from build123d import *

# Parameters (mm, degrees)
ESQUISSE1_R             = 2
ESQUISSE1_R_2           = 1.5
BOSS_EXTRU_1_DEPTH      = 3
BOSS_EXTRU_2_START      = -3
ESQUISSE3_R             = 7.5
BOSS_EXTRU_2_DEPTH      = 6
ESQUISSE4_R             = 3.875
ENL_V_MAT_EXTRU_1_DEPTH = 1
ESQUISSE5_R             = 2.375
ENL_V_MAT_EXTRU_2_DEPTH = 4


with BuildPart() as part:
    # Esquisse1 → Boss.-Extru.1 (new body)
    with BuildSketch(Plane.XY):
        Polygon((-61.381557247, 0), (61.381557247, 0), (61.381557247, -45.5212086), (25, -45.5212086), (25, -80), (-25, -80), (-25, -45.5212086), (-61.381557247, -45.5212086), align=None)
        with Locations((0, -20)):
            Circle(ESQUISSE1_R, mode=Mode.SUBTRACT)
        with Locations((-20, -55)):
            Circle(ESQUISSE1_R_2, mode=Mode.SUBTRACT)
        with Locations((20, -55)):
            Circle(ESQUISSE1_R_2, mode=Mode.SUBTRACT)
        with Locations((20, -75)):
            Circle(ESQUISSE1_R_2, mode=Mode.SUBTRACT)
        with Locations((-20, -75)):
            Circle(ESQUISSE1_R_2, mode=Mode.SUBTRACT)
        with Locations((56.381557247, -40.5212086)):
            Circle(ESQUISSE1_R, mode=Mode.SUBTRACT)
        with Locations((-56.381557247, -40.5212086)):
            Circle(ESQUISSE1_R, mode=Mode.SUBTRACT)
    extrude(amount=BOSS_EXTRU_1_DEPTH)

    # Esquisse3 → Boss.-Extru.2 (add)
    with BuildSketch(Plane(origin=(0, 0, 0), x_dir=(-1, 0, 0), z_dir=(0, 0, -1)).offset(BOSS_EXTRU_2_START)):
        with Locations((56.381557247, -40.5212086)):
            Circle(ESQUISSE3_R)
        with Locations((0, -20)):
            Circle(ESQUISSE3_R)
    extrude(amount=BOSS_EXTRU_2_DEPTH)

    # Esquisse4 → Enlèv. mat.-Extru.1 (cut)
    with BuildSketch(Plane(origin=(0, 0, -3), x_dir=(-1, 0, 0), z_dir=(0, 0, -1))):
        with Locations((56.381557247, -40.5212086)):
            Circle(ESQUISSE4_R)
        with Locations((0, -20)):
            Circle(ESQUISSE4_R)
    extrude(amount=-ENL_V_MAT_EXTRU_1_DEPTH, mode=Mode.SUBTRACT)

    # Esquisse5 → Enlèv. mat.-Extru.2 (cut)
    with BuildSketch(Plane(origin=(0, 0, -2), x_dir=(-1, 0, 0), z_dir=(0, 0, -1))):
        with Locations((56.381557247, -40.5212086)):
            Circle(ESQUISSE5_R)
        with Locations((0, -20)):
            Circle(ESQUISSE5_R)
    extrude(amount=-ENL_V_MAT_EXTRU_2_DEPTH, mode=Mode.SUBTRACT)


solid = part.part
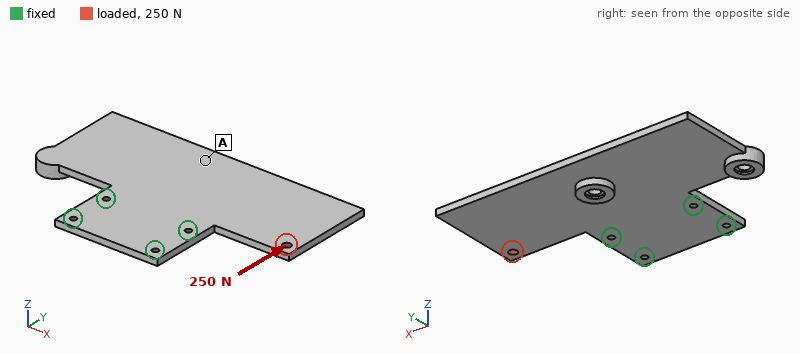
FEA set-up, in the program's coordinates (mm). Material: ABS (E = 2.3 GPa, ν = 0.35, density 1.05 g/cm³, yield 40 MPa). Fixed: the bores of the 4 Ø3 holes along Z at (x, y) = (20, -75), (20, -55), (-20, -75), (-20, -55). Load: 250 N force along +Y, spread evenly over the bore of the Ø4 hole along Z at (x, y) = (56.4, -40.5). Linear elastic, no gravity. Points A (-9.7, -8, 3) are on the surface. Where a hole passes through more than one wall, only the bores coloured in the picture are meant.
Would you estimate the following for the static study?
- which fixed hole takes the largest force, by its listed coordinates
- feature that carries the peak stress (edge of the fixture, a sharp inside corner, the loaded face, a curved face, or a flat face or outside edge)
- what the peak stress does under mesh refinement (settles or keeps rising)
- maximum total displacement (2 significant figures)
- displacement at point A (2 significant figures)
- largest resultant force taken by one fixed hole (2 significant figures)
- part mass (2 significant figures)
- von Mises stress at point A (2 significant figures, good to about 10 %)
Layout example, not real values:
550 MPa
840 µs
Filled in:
(20, -55)
edge of the fixture
keeps rising
0.66 mm
0.22 mm
410 N
24 g
2.8 MPa
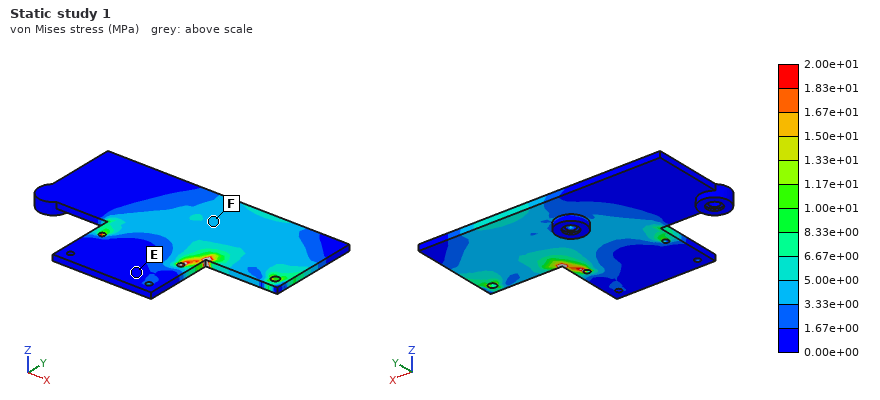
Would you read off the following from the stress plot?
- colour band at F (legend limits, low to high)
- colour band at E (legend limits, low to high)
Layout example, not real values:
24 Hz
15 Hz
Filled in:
3.33e+00 to 5.00e+00 MPa
0.00e+00 to 1.67e+00 MPa
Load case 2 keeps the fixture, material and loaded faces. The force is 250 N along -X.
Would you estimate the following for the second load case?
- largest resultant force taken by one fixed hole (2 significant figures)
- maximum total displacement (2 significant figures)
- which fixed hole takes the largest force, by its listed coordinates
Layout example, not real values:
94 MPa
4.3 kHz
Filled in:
160 N
0.18 mm
(20, -55)
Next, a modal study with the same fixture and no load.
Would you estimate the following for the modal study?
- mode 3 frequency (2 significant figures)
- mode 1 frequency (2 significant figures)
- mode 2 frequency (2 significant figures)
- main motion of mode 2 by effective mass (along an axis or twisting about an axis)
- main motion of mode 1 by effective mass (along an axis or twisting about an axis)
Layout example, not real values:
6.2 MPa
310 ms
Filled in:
310 Hz
150 Hz
170 Hz
twisting about Y
along Z
